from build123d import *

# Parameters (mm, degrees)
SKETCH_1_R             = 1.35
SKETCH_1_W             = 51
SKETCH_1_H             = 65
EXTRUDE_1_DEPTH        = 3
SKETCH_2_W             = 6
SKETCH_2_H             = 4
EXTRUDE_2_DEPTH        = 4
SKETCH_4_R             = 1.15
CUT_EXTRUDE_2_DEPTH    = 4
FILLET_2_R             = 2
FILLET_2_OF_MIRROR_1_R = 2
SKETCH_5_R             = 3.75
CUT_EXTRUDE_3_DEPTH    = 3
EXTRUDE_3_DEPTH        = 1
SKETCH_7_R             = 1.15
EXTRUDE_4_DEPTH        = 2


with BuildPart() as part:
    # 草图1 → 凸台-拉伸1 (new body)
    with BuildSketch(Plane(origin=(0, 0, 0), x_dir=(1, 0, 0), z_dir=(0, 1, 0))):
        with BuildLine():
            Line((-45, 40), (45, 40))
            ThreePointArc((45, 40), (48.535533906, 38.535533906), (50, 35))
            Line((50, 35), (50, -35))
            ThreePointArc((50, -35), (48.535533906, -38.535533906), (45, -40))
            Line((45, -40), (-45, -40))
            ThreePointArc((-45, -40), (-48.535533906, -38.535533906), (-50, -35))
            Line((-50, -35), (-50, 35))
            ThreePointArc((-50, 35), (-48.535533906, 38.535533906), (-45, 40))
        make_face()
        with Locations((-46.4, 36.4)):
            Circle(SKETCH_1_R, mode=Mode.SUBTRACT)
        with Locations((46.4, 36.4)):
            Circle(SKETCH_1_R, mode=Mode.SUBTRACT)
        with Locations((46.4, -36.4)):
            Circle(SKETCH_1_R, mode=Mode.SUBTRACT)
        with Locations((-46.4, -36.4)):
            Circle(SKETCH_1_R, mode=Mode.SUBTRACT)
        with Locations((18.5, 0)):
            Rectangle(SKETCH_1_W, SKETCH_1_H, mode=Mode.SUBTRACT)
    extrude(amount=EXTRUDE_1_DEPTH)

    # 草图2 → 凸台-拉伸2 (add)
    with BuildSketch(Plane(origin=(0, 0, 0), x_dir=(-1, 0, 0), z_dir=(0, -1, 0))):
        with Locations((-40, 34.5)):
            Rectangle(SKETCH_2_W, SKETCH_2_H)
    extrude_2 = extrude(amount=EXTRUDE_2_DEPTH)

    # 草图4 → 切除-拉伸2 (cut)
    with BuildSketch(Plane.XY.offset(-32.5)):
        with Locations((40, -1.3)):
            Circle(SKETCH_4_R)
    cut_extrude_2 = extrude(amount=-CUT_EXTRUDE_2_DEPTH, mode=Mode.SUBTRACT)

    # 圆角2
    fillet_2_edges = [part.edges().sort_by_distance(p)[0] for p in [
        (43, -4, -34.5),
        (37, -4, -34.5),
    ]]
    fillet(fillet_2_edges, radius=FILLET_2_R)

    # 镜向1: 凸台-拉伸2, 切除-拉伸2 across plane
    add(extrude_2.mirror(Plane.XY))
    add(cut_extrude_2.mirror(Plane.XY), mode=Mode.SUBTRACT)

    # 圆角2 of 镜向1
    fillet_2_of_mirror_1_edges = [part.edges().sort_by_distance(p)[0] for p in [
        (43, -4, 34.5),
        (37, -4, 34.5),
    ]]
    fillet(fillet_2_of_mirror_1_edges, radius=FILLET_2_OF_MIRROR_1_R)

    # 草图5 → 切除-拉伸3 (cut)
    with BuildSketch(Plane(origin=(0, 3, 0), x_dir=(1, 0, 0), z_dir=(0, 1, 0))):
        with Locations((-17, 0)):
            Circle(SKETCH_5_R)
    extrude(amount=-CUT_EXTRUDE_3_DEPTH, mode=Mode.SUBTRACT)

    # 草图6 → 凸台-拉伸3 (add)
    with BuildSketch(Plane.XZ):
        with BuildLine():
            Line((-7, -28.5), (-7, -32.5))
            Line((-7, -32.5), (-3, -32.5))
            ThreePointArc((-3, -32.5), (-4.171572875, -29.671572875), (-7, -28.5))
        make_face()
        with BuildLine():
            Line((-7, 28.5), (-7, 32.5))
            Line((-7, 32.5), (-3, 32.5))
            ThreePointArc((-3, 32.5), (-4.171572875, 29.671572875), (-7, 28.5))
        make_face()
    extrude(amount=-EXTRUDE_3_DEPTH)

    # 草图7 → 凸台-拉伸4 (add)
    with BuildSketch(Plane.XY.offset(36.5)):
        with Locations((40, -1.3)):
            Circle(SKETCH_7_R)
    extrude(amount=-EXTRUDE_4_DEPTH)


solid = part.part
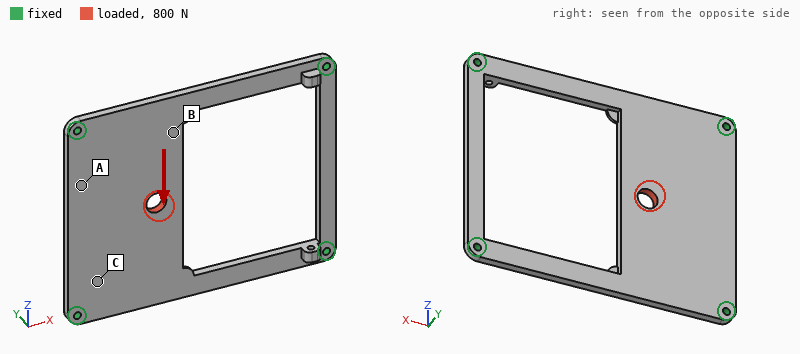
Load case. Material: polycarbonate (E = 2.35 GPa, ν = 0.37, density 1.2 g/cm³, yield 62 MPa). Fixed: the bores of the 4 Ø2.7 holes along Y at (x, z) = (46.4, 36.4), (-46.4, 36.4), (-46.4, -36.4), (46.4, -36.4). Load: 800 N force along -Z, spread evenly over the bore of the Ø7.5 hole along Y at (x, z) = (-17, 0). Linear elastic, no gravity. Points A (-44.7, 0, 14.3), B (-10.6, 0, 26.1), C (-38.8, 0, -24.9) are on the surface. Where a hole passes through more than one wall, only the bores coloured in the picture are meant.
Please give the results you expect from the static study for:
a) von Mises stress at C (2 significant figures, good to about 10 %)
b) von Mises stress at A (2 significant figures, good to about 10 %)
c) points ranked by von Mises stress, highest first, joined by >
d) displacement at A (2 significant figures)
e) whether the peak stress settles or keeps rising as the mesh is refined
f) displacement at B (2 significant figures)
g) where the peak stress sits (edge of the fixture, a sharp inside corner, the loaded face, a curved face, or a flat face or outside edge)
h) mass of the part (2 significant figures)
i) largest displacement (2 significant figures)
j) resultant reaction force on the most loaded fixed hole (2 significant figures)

8.4 MPa
4.4 MPa
C > A > B
0.083 mm
keeps rising
0.21 mm
edge of the fixture
17 g
0.27 mm
480 N
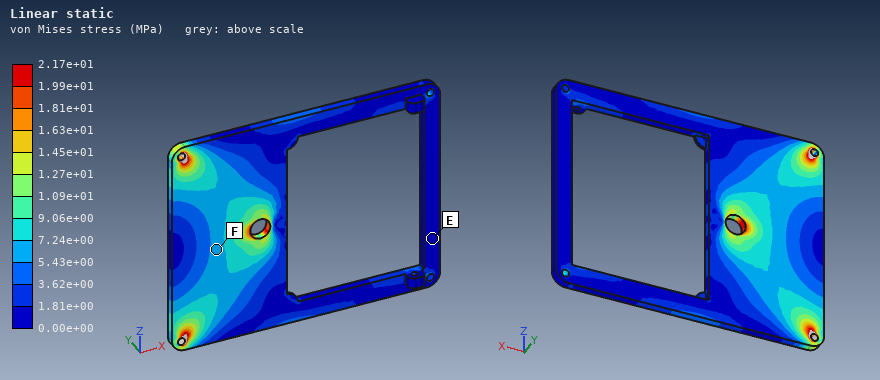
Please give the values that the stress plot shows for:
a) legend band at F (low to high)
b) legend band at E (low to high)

5.43e+00 to 7.24e+00 MPa
0.00e+00 to 1.81e+00 MPa
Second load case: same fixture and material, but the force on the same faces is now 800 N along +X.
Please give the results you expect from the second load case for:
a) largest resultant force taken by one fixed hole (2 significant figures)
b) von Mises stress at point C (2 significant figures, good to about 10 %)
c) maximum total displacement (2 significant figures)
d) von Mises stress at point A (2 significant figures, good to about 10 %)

430 N
9.0 MPa
0.31 mm
3.9 MPa
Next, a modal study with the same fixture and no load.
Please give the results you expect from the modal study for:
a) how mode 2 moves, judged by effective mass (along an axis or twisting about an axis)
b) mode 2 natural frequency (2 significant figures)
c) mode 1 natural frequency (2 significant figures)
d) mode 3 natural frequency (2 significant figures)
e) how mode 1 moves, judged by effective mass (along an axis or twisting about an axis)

twisting about X
580 Hz
350 Hz
730 Hz
along Y
